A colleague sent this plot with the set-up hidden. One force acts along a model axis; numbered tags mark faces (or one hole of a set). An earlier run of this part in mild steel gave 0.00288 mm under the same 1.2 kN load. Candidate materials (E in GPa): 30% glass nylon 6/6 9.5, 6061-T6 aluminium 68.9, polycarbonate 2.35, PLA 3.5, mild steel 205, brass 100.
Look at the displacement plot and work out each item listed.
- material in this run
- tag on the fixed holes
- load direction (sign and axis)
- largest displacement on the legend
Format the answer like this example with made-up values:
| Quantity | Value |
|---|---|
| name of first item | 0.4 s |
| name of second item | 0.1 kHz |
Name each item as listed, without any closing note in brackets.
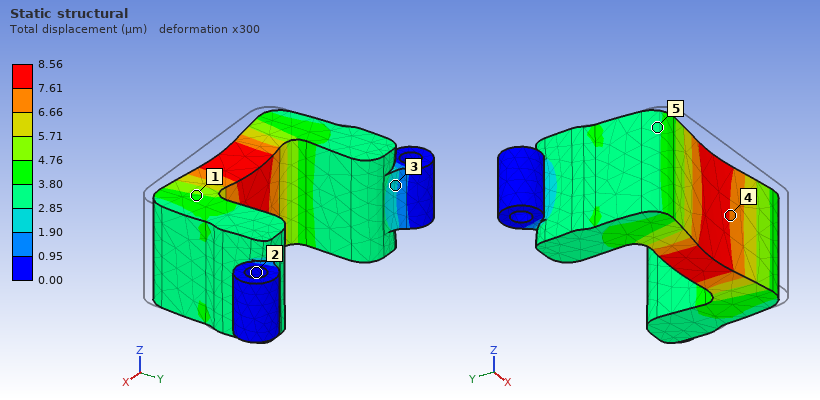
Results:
| Quantity | Value |
|---|---|
| material in this run | 6061-T6 aluminium |
| tag on the fixed holes | 2 |
| load direction | +Y |
| largest displacement on the legend | 8.56 µm |
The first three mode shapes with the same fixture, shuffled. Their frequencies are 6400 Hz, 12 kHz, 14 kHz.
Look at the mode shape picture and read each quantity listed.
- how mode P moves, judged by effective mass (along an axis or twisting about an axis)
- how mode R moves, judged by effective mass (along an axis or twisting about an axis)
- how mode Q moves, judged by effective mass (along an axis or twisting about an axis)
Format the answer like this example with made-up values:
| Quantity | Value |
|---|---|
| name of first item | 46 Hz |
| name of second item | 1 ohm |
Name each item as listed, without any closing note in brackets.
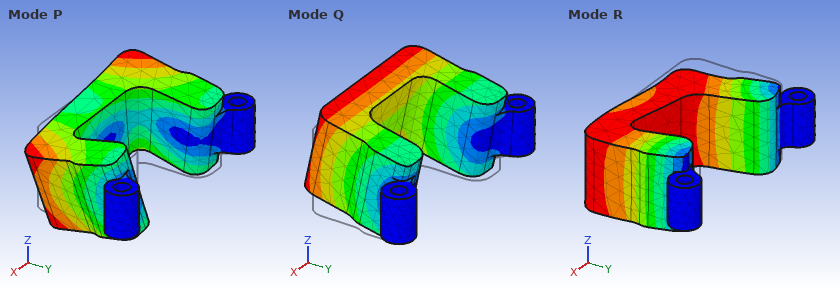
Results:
| Quantity | Value |
|---|---|
| how mode P moves, judged by effective mass | twisting about Y |
| how mode R moves, judged by effective mass | along X |
| how mode Q moves, judged by effective mass | along Z |
